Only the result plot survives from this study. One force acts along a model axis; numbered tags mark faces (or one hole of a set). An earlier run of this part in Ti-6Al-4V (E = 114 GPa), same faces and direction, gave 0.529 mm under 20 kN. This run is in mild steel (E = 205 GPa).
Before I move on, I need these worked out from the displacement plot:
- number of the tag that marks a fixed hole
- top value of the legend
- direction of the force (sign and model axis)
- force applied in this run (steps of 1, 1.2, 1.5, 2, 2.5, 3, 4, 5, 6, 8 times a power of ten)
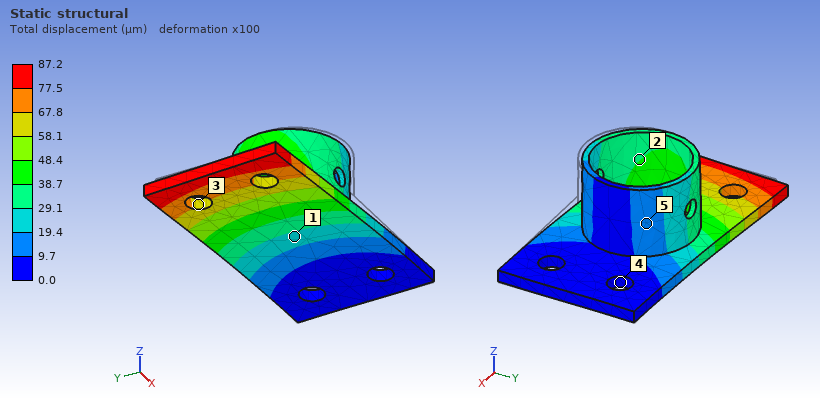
4
87.2 µm
+Y
6 kN
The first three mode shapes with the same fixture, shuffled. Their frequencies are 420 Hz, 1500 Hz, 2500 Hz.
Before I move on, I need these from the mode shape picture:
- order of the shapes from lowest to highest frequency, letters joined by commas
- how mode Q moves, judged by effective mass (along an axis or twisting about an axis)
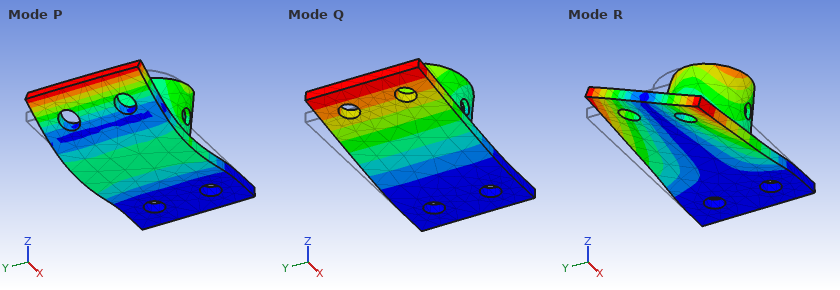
Q, R, P
along Z
